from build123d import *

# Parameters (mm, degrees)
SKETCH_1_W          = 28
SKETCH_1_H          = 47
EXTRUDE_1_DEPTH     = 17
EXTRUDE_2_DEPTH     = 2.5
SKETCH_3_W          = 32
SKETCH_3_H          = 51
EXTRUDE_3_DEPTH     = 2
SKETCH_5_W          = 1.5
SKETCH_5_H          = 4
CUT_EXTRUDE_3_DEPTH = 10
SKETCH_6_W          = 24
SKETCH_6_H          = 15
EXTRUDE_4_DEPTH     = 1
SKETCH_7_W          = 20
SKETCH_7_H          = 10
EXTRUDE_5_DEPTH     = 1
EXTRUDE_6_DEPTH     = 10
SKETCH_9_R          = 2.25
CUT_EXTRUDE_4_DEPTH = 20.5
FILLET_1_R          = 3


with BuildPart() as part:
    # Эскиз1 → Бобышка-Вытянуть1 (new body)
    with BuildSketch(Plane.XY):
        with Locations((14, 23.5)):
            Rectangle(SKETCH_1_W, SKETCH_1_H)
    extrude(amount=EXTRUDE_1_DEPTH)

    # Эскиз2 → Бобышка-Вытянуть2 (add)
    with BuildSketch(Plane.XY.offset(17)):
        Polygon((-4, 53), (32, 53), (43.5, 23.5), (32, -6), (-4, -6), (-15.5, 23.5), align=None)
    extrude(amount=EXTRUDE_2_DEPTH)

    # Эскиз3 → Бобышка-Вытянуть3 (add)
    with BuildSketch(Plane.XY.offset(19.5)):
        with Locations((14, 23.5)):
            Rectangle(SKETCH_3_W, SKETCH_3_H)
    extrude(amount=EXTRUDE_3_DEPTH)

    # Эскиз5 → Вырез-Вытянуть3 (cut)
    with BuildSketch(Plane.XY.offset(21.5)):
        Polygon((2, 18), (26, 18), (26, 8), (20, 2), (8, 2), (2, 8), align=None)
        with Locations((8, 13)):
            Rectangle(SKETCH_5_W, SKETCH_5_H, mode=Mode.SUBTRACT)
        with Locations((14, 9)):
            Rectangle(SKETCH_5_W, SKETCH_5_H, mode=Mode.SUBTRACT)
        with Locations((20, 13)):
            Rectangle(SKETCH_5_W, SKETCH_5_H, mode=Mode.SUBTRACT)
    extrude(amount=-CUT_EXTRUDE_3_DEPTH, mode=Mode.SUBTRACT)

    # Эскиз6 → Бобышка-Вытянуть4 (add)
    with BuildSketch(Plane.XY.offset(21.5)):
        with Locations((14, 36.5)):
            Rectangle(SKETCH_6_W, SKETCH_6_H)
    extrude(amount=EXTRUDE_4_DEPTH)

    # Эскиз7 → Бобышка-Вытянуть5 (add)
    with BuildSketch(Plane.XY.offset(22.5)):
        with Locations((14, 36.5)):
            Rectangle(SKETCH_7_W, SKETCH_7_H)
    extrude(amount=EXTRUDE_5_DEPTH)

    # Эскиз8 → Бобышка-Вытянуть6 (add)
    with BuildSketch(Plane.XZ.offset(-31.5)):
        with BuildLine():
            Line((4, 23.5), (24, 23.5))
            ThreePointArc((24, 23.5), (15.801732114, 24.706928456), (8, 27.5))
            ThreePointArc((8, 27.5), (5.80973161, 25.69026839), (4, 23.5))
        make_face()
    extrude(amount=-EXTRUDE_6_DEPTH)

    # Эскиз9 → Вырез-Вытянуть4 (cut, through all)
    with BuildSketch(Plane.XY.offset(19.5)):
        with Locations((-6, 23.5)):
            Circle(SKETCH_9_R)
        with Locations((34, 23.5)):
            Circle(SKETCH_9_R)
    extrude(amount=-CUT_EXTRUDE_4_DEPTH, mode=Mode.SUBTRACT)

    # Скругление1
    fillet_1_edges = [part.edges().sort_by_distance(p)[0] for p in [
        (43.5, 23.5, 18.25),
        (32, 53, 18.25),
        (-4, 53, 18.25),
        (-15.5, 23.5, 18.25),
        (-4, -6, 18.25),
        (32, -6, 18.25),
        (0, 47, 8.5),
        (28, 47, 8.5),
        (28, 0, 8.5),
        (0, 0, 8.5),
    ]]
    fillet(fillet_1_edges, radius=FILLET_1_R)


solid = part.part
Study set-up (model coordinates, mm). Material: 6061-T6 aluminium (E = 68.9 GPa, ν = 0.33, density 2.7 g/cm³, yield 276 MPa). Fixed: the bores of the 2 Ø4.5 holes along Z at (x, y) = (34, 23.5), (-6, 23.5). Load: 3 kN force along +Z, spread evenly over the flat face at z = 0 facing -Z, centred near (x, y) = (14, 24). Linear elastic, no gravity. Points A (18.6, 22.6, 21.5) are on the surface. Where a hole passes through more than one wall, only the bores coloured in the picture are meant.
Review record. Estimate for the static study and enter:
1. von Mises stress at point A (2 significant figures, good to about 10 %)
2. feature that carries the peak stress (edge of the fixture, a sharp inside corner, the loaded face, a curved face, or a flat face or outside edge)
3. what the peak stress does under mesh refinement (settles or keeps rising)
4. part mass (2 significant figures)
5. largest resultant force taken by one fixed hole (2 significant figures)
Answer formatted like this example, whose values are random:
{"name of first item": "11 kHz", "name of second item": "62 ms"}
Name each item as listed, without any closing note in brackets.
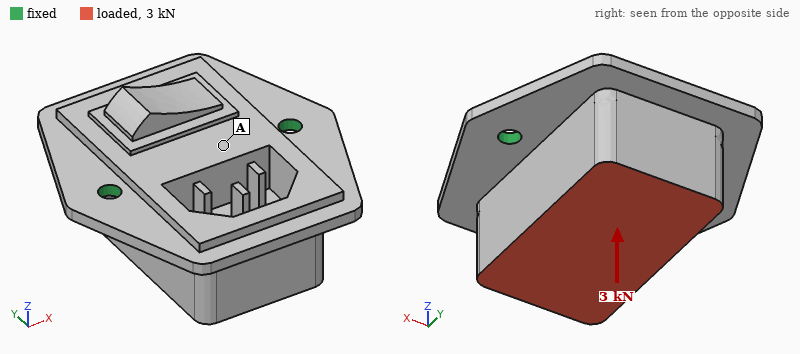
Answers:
{"von Mises stress at point A": "19 MPa", "feature that carries the peak stress": "edge of the fixture", "what the peak stress does under mesh refinement": "keeps rising", "part mass": "81 g", "largest resultant force taken by one fixed hole": "1.5 kN"}
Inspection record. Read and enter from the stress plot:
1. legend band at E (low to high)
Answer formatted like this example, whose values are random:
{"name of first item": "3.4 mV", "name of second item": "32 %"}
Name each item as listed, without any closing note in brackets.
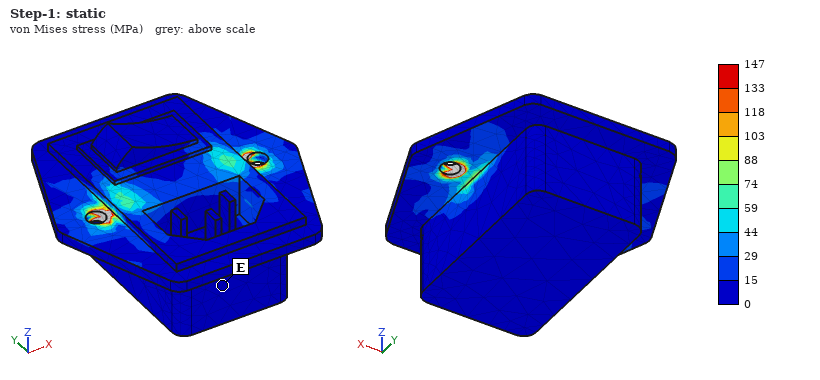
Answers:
{"legend band at E": "0 to 15 MPa"}
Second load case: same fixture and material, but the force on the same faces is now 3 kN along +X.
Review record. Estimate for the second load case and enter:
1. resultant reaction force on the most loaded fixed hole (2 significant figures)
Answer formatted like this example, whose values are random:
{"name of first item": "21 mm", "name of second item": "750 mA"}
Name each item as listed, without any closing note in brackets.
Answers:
{"resultant reaction force on the most loaded fixed hole": "2.2 kN"}
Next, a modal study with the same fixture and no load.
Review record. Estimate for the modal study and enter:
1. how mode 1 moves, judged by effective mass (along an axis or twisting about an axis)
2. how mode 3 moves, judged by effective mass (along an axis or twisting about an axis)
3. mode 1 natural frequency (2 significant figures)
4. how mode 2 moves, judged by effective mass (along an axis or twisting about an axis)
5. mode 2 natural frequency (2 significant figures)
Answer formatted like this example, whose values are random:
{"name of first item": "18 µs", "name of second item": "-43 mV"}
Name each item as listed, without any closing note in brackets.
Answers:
{"how mode 1 moves, judged by effective mass": "along Y", "how mode 3 moves, judged by effective mass": "along X", "mode 1 natural frequency": "1500 Hz", "how mode 2 moves, judged by effective mass": "along Z", "mode 2 natural frequency": "6100 Hz"}
